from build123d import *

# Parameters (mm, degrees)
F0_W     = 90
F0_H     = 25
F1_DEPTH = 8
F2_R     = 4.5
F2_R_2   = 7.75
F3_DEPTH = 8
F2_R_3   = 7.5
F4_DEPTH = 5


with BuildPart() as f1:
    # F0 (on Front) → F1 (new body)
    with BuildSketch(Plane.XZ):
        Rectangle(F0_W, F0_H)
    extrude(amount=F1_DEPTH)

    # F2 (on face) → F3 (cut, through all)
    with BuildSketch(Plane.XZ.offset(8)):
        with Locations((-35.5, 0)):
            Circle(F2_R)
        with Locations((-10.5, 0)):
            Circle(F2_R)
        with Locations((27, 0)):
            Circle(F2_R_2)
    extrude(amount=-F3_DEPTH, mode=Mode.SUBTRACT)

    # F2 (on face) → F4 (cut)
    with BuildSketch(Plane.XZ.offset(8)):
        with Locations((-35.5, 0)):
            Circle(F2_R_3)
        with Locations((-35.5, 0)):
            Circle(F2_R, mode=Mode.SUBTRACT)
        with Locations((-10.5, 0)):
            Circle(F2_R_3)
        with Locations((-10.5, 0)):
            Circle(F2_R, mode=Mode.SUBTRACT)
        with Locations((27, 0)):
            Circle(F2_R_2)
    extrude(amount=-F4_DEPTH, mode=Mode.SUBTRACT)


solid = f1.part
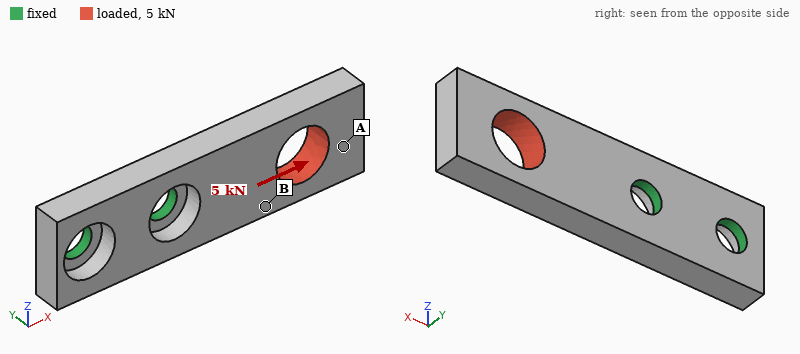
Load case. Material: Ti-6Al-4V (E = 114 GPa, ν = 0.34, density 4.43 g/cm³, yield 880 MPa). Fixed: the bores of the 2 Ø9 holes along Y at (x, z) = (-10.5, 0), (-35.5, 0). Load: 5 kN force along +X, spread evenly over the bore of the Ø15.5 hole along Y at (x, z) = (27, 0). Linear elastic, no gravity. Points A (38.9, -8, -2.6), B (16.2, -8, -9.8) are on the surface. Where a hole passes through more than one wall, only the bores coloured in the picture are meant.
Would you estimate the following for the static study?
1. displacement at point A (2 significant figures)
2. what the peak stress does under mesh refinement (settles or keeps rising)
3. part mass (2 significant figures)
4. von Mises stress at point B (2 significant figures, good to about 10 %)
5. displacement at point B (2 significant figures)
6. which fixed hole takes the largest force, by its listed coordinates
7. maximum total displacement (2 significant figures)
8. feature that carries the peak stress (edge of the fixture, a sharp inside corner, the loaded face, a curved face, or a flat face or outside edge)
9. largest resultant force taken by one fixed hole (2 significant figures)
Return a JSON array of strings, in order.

["60 µm", "keeps rising", "64 g", "35 MPa", "33 µm", "(-10.5, 0)", "67 µm", "edge of the fixture", "3.7 kN"]
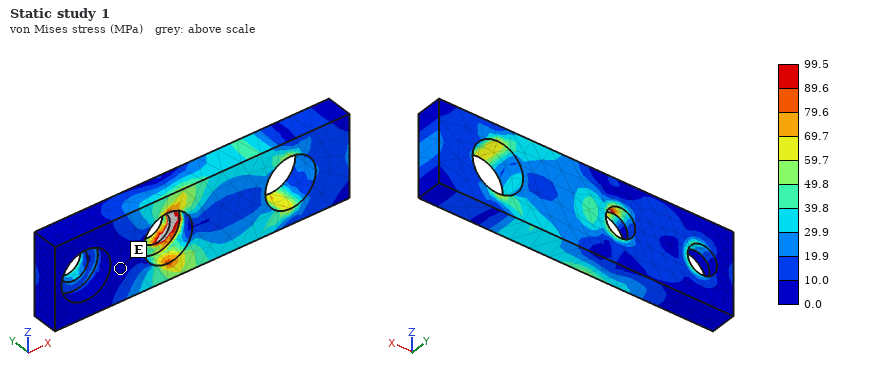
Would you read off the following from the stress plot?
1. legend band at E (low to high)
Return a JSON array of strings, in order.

["0.0 to 10.0 MPa"]
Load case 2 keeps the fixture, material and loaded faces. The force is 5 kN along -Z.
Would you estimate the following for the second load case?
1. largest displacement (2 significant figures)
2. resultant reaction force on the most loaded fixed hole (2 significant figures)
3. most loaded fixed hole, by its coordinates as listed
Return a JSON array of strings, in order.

["0.31 mm", "9.0 kN", "(-10.5, 0)"]
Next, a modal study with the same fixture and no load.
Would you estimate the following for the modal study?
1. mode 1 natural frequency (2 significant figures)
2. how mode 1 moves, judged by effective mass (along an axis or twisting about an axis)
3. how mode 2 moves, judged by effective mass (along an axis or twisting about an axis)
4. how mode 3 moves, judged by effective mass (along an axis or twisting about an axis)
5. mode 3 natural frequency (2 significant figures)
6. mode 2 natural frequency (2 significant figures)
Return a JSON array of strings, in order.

["1900 Hz", "along Y", "along Z", "twisting about X", "6200 Hz", "4600 Hz"]
